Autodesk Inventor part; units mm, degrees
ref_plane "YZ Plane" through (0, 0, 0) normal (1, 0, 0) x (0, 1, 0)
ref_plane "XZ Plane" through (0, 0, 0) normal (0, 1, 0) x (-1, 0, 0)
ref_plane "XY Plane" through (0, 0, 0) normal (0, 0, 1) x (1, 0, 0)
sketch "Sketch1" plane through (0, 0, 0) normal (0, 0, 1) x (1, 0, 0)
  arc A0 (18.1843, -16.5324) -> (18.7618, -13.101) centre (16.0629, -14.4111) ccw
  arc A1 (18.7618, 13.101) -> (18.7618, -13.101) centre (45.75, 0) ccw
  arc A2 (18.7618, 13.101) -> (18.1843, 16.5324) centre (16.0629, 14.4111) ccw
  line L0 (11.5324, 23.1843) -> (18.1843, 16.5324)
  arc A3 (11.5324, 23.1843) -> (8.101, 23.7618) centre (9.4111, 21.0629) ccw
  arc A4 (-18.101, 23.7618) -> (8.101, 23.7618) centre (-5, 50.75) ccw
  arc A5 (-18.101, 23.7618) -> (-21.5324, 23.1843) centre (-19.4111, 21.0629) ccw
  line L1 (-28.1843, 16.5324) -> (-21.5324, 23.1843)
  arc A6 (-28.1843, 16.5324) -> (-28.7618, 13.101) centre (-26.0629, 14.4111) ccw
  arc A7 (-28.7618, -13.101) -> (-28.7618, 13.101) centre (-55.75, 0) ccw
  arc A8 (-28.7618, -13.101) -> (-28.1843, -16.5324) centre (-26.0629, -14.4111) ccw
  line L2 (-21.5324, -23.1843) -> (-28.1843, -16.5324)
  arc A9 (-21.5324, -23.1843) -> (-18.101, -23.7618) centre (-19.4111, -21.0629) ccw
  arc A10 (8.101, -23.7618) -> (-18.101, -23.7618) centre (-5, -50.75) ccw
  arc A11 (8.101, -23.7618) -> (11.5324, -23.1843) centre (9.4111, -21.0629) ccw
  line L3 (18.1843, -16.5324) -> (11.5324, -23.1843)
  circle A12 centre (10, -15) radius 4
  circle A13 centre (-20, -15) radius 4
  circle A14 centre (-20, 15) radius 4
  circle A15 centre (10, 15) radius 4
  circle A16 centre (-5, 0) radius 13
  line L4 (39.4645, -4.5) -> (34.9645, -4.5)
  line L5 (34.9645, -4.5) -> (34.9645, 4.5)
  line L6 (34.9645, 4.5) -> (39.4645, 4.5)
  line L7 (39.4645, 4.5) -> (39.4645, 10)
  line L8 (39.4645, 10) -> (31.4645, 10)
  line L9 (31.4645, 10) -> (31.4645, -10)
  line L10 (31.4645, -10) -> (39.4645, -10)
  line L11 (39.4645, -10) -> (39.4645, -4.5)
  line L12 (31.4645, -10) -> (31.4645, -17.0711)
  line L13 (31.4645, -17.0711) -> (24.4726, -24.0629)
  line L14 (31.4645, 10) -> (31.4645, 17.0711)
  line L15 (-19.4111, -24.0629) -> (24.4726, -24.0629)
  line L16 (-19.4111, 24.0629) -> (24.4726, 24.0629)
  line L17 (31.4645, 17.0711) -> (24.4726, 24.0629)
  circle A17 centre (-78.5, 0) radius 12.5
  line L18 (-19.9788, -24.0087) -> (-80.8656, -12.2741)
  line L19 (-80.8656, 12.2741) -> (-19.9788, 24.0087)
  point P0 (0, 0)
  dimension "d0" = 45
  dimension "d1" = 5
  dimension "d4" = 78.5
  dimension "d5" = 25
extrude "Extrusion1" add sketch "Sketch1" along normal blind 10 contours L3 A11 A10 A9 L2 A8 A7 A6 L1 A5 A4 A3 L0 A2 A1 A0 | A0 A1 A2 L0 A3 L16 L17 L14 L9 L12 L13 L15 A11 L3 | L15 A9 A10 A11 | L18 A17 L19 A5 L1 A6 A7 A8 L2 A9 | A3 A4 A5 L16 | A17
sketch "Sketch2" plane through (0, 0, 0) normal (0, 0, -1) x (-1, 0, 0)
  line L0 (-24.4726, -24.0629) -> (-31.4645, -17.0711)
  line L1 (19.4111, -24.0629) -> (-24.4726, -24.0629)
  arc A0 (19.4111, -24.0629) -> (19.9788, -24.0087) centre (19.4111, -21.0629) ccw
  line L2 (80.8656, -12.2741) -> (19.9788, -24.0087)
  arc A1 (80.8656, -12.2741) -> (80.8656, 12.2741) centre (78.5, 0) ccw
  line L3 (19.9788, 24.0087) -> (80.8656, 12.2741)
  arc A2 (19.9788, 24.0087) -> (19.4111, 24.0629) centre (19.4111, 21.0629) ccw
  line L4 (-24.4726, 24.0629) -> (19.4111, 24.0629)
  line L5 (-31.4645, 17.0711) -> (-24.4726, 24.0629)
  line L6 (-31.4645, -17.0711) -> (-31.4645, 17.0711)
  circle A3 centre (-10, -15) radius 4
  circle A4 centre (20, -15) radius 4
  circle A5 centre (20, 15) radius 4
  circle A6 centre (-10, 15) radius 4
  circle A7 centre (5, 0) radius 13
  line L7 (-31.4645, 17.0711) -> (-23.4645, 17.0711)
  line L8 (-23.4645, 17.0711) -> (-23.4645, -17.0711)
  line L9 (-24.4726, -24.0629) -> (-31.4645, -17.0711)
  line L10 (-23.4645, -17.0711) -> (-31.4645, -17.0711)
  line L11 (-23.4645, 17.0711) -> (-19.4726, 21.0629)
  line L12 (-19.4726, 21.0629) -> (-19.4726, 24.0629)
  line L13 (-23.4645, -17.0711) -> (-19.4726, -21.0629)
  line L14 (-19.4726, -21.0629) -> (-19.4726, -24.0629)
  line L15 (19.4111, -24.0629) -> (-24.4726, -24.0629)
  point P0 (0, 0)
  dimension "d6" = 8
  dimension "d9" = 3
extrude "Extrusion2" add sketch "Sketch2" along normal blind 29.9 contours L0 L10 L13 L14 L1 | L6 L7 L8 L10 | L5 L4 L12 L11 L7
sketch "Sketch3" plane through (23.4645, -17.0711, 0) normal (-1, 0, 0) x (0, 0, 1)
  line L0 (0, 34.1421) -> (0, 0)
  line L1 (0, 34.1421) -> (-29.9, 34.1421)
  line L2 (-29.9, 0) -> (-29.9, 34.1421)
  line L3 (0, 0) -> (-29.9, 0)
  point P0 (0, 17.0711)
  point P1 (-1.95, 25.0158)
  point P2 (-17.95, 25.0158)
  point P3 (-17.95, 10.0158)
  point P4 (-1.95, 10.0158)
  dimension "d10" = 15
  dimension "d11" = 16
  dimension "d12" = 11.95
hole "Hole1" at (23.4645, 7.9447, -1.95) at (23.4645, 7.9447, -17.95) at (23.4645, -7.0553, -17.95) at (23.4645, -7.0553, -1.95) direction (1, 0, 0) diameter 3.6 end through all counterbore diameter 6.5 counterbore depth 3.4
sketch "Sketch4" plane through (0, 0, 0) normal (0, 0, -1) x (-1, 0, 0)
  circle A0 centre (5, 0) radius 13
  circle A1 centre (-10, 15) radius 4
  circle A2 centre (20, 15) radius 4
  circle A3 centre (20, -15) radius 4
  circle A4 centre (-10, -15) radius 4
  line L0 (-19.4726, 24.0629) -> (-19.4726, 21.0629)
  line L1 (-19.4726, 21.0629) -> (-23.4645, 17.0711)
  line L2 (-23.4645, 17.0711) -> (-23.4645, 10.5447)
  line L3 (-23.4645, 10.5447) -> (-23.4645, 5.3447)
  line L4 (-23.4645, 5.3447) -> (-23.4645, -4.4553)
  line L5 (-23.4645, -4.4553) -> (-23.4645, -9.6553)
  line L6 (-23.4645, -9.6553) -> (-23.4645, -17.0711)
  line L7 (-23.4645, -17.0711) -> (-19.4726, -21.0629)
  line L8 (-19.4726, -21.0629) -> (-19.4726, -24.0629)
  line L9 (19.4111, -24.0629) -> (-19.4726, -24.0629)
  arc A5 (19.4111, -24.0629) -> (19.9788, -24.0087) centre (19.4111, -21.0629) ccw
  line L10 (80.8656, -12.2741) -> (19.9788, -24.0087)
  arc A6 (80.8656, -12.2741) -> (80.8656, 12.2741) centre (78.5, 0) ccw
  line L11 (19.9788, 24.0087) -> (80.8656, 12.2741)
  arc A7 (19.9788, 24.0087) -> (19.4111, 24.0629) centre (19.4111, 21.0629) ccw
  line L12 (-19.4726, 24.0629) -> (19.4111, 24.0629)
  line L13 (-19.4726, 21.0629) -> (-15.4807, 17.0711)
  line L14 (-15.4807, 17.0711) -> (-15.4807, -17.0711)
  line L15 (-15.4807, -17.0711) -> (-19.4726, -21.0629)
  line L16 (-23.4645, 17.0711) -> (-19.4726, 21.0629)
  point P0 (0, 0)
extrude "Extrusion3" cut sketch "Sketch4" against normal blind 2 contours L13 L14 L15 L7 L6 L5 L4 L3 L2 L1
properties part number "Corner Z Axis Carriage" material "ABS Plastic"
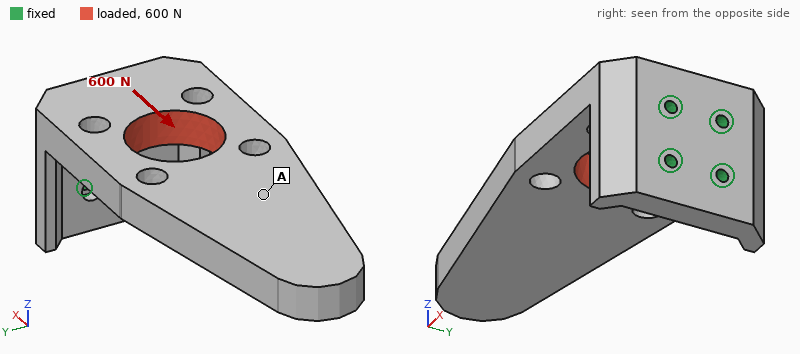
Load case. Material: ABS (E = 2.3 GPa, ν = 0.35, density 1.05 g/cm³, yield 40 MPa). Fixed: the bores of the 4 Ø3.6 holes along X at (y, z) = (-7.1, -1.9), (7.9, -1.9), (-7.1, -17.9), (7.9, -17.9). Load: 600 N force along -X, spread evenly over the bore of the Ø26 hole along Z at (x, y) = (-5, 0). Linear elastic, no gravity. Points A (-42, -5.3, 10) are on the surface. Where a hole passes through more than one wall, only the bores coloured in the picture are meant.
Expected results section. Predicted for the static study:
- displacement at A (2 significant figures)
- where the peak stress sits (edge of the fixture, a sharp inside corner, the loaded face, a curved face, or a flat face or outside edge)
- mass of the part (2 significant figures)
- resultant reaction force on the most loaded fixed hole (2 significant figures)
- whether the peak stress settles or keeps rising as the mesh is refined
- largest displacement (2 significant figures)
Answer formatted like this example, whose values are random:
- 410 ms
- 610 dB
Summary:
- 0.50 mm
- edge of the fixture
- 53 g
- 390 N
- keeps rising
- 0.82 mm
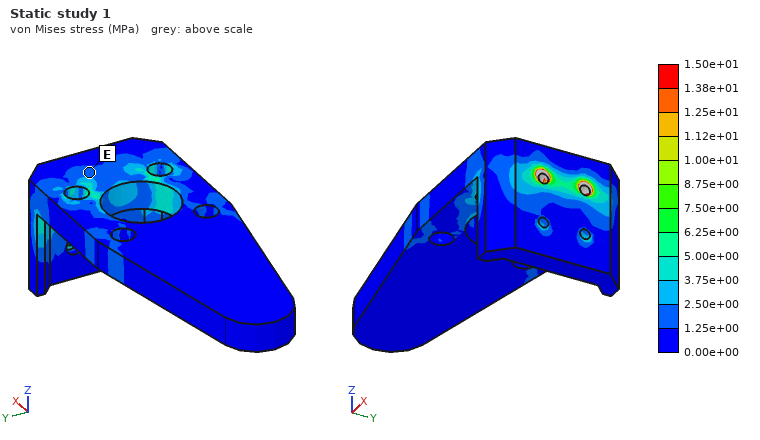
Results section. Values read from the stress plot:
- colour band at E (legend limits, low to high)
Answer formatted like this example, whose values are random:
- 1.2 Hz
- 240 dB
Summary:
- 1.25e+00 to 2.50e+00 MPa
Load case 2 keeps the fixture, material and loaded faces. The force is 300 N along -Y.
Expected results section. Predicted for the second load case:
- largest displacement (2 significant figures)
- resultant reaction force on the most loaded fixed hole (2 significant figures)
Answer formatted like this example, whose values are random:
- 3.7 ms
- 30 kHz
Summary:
- 1.2 mm
- 510 N
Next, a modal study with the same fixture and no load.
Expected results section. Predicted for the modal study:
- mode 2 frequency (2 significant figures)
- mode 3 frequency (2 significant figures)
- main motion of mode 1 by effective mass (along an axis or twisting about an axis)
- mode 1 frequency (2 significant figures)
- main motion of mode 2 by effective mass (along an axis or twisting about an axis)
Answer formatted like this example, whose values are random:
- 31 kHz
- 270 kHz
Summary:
- 360 Hz
- 910 Hz
- along Z
- 140 Hz
- along Y
